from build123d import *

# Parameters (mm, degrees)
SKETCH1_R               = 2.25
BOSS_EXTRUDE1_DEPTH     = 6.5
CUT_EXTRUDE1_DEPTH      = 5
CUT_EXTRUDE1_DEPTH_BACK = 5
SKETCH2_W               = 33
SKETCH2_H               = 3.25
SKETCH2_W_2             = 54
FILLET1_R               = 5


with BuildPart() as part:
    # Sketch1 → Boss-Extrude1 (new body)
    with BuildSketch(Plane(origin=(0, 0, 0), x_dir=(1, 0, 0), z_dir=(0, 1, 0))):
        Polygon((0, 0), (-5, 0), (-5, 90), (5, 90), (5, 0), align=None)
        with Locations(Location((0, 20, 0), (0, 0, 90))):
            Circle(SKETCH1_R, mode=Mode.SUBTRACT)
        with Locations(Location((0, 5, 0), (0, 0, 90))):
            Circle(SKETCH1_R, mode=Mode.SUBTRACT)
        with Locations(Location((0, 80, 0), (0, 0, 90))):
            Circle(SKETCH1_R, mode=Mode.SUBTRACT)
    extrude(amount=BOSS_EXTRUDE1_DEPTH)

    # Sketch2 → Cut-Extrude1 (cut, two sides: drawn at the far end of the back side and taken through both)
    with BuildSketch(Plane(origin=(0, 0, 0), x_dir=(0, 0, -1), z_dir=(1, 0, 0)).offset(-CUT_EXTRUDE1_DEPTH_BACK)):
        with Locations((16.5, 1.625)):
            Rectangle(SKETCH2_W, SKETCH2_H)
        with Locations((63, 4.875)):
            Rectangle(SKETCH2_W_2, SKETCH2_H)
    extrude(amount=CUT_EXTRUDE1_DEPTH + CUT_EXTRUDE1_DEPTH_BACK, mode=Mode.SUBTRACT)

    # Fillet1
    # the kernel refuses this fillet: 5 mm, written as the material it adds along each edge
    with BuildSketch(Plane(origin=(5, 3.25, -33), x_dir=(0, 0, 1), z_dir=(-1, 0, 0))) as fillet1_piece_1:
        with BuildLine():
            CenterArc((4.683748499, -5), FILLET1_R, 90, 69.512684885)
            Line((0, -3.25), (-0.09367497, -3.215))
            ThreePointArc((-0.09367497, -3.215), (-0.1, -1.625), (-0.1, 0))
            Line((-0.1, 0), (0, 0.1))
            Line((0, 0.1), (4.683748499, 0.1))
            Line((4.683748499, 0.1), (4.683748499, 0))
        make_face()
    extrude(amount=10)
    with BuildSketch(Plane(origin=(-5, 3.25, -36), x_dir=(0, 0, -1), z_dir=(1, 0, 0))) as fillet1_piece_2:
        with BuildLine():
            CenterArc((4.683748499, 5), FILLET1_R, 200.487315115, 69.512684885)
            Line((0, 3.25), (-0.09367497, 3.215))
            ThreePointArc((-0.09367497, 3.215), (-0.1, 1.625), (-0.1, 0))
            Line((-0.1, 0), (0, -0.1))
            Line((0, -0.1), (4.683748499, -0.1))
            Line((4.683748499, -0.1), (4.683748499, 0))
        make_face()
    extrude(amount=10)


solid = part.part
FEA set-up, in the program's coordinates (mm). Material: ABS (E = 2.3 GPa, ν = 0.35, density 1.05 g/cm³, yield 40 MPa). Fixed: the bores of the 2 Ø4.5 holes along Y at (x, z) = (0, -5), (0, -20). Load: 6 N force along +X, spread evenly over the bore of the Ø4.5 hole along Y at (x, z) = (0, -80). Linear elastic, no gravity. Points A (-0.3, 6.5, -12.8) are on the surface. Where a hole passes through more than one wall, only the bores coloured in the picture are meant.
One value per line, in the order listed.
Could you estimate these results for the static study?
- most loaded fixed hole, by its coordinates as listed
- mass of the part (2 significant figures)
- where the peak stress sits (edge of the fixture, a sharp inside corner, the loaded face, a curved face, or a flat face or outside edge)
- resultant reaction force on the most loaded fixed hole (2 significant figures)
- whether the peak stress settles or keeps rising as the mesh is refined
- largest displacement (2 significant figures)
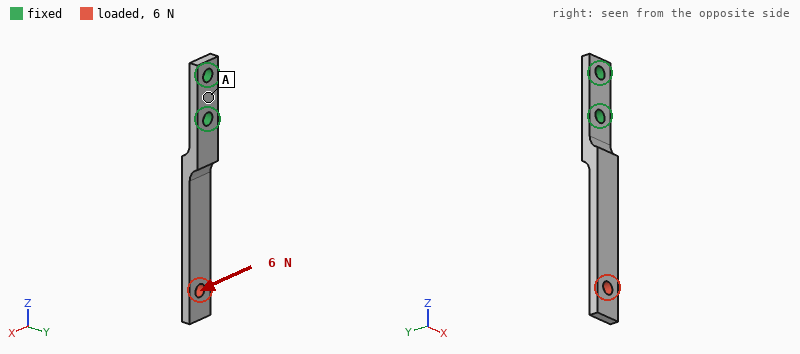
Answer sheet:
(0, -20)
3.1 g
edge of the fixture
12 N
keeps rising
0.93 mm
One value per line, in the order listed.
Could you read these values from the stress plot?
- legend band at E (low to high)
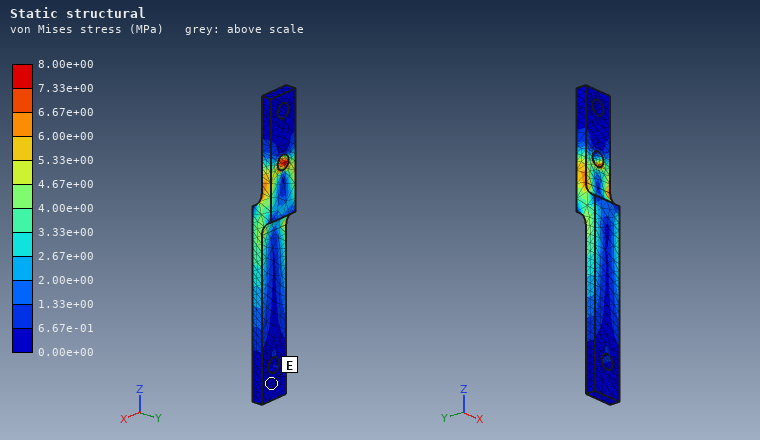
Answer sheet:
0.00e+00 to 6.67e-01 MPa
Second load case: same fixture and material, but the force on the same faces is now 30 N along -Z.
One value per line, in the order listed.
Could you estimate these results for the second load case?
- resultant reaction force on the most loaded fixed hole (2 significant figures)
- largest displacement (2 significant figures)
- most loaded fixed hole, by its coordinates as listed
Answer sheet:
29 N
0.95 mm
(0, -20)
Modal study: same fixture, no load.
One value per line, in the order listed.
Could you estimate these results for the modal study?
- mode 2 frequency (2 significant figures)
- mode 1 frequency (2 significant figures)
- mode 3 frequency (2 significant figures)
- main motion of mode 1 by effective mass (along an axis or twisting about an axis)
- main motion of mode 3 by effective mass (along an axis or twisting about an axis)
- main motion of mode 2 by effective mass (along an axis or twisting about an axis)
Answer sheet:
480 Hz
190 Hz
1000 Hz
along Y
along Y
along X
